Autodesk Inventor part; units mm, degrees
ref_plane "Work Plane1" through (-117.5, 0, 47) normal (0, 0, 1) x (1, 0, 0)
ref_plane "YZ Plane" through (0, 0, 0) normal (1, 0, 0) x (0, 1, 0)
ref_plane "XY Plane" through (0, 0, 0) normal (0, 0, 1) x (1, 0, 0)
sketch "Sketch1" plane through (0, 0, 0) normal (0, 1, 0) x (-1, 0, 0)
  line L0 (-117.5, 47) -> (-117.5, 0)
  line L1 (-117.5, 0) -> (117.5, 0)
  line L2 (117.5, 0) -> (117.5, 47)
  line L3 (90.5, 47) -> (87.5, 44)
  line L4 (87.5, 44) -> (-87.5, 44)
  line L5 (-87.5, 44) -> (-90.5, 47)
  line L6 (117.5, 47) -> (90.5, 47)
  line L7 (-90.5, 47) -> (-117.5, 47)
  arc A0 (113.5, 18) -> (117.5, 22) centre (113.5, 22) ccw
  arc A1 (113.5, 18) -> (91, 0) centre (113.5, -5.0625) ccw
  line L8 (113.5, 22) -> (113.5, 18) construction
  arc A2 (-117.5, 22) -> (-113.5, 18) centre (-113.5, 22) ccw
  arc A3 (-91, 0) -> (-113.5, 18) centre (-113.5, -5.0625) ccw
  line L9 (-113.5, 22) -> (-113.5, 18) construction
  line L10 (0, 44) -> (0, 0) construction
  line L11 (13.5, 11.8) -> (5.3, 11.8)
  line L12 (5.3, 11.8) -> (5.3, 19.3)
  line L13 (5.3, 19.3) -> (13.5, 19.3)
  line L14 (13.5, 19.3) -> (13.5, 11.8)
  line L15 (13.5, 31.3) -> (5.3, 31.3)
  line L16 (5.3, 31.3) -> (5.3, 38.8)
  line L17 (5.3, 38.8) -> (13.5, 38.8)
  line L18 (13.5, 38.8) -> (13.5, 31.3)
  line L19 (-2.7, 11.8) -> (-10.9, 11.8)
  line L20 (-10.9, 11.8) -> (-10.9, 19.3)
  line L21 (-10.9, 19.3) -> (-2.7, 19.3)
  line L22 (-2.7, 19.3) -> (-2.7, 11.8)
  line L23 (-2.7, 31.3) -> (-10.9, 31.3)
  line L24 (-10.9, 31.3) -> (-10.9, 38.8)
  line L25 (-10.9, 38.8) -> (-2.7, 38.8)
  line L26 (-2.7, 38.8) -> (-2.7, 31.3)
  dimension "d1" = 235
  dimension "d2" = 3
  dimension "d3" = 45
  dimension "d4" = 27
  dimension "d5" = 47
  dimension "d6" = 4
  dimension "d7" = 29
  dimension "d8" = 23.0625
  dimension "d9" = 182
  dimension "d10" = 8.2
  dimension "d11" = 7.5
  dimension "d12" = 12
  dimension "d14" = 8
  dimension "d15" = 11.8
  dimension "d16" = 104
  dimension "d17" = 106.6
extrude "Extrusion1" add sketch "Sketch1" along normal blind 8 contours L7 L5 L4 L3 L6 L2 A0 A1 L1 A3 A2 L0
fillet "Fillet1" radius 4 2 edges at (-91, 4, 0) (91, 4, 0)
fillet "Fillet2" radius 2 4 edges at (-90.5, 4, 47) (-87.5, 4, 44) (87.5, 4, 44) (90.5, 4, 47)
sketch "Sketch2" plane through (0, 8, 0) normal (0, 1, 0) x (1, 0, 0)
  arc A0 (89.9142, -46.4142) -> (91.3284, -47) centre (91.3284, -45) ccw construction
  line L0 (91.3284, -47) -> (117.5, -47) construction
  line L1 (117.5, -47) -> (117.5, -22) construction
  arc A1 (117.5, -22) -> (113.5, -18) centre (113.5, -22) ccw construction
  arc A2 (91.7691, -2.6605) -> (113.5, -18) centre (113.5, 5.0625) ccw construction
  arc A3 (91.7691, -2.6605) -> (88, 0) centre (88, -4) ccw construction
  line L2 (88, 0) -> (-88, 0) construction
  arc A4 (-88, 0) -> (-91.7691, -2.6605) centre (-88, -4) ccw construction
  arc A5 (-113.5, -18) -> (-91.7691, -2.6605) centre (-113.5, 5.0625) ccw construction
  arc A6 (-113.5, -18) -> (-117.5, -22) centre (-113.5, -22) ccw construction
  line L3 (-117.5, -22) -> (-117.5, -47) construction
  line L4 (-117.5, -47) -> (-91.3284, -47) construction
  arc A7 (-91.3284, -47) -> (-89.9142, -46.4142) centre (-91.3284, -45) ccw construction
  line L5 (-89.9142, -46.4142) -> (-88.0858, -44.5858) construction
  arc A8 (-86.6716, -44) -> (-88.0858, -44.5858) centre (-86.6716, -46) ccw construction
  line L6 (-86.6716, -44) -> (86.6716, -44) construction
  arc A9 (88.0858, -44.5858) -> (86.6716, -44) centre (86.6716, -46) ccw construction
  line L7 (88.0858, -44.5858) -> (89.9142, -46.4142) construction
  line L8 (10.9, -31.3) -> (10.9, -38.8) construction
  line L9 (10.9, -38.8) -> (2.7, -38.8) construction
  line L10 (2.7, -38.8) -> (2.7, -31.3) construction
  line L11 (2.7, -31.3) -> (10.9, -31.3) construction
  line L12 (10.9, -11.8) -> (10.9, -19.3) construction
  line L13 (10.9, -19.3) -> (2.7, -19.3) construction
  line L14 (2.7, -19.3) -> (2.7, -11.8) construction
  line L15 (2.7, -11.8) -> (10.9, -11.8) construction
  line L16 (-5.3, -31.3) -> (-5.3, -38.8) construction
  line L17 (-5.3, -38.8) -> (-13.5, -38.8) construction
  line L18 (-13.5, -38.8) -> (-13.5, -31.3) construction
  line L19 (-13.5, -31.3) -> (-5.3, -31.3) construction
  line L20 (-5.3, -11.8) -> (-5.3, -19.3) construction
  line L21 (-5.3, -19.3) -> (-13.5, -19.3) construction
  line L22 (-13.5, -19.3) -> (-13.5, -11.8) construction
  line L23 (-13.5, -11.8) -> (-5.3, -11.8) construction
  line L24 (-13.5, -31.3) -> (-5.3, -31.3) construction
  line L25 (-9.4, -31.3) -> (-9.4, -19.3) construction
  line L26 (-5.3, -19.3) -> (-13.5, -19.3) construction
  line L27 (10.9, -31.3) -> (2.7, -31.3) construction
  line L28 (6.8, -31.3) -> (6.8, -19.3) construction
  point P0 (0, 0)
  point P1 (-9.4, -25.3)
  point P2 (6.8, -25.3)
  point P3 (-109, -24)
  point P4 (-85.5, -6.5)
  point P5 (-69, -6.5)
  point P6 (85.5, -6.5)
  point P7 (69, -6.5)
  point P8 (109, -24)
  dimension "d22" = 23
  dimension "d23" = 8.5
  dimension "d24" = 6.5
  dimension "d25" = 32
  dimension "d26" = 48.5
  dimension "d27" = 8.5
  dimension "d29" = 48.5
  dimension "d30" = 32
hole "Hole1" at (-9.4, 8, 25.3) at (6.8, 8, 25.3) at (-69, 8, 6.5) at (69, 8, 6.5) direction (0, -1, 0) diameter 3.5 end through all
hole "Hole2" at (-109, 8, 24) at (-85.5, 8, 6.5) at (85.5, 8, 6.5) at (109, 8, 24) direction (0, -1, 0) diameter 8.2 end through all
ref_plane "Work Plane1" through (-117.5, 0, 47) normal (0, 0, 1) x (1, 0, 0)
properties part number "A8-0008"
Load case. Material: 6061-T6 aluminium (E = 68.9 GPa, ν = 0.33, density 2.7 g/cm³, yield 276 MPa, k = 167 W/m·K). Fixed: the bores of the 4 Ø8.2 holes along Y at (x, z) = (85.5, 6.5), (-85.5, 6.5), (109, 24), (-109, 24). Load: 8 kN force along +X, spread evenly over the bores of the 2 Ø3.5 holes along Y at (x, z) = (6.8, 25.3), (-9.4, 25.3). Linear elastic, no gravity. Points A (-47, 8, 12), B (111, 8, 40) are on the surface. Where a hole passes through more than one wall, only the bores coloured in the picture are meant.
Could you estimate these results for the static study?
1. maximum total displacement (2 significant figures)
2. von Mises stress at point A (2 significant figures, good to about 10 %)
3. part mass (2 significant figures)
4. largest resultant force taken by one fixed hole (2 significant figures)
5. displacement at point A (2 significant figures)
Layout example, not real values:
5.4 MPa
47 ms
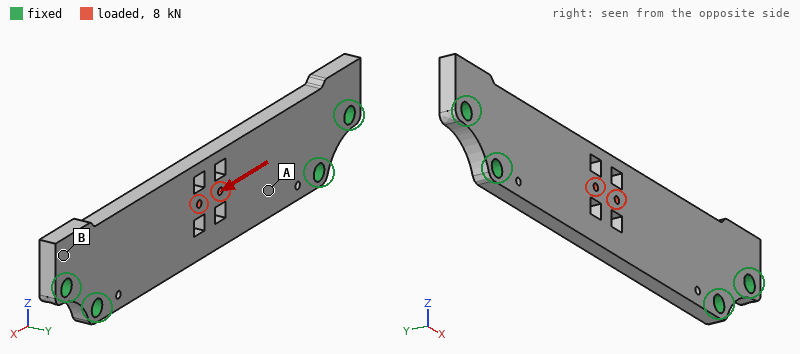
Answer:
22 µm
13 MPa
200 g
2.4 kN
8.6 µm
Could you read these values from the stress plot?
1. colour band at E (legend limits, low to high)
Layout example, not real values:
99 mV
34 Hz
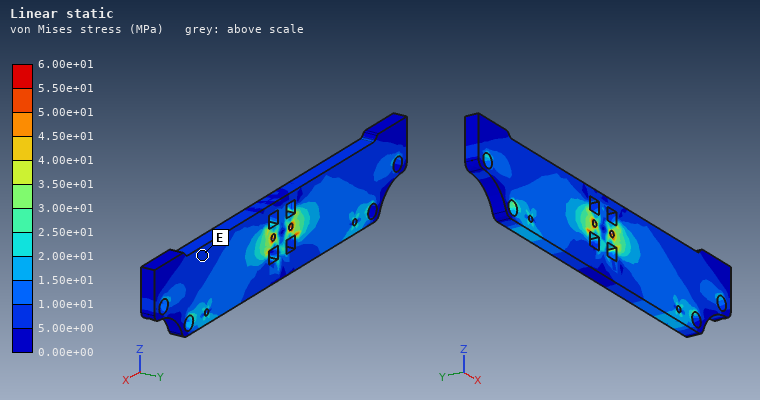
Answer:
5.00e+00 to 1.00e+01 MPa
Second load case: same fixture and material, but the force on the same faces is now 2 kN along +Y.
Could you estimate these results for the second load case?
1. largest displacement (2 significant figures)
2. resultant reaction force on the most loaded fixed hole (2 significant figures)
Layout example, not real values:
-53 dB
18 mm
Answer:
0.62 mm
1.4 kN
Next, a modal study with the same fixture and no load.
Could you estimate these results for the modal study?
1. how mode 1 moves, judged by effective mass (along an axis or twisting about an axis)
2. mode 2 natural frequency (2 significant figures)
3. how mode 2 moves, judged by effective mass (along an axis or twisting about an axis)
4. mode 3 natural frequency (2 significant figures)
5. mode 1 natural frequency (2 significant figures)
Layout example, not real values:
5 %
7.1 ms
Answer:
along Y
3100 Hz
twisting about X
3300 Hz
1300 Hz
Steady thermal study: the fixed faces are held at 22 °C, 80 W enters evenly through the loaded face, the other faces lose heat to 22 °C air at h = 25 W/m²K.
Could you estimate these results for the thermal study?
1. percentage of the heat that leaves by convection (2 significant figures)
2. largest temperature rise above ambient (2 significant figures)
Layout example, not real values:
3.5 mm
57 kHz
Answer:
17 %
64 K
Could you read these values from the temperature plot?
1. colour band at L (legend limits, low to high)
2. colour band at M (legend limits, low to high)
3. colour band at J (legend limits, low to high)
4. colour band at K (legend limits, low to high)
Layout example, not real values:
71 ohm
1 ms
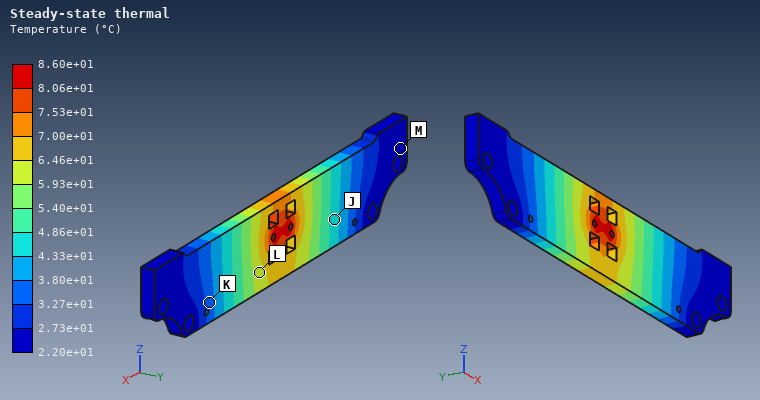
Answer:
5.93e+01 to 6.46e+01 °C
2.20e+01 to 2.73e+01 °C
4.33e+01 to 4.86e+01 °C
3.27e+01 to 3.80e+01 °C
